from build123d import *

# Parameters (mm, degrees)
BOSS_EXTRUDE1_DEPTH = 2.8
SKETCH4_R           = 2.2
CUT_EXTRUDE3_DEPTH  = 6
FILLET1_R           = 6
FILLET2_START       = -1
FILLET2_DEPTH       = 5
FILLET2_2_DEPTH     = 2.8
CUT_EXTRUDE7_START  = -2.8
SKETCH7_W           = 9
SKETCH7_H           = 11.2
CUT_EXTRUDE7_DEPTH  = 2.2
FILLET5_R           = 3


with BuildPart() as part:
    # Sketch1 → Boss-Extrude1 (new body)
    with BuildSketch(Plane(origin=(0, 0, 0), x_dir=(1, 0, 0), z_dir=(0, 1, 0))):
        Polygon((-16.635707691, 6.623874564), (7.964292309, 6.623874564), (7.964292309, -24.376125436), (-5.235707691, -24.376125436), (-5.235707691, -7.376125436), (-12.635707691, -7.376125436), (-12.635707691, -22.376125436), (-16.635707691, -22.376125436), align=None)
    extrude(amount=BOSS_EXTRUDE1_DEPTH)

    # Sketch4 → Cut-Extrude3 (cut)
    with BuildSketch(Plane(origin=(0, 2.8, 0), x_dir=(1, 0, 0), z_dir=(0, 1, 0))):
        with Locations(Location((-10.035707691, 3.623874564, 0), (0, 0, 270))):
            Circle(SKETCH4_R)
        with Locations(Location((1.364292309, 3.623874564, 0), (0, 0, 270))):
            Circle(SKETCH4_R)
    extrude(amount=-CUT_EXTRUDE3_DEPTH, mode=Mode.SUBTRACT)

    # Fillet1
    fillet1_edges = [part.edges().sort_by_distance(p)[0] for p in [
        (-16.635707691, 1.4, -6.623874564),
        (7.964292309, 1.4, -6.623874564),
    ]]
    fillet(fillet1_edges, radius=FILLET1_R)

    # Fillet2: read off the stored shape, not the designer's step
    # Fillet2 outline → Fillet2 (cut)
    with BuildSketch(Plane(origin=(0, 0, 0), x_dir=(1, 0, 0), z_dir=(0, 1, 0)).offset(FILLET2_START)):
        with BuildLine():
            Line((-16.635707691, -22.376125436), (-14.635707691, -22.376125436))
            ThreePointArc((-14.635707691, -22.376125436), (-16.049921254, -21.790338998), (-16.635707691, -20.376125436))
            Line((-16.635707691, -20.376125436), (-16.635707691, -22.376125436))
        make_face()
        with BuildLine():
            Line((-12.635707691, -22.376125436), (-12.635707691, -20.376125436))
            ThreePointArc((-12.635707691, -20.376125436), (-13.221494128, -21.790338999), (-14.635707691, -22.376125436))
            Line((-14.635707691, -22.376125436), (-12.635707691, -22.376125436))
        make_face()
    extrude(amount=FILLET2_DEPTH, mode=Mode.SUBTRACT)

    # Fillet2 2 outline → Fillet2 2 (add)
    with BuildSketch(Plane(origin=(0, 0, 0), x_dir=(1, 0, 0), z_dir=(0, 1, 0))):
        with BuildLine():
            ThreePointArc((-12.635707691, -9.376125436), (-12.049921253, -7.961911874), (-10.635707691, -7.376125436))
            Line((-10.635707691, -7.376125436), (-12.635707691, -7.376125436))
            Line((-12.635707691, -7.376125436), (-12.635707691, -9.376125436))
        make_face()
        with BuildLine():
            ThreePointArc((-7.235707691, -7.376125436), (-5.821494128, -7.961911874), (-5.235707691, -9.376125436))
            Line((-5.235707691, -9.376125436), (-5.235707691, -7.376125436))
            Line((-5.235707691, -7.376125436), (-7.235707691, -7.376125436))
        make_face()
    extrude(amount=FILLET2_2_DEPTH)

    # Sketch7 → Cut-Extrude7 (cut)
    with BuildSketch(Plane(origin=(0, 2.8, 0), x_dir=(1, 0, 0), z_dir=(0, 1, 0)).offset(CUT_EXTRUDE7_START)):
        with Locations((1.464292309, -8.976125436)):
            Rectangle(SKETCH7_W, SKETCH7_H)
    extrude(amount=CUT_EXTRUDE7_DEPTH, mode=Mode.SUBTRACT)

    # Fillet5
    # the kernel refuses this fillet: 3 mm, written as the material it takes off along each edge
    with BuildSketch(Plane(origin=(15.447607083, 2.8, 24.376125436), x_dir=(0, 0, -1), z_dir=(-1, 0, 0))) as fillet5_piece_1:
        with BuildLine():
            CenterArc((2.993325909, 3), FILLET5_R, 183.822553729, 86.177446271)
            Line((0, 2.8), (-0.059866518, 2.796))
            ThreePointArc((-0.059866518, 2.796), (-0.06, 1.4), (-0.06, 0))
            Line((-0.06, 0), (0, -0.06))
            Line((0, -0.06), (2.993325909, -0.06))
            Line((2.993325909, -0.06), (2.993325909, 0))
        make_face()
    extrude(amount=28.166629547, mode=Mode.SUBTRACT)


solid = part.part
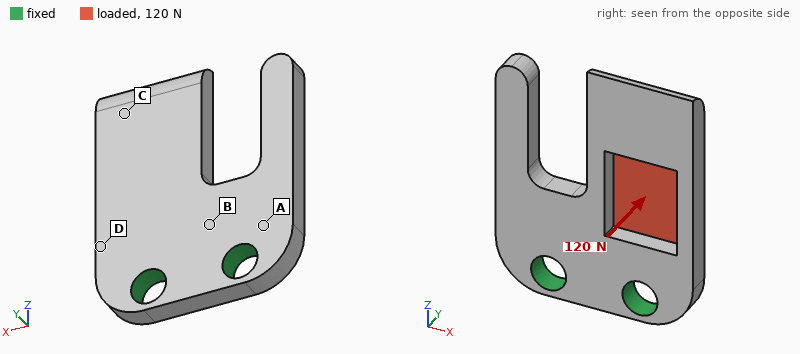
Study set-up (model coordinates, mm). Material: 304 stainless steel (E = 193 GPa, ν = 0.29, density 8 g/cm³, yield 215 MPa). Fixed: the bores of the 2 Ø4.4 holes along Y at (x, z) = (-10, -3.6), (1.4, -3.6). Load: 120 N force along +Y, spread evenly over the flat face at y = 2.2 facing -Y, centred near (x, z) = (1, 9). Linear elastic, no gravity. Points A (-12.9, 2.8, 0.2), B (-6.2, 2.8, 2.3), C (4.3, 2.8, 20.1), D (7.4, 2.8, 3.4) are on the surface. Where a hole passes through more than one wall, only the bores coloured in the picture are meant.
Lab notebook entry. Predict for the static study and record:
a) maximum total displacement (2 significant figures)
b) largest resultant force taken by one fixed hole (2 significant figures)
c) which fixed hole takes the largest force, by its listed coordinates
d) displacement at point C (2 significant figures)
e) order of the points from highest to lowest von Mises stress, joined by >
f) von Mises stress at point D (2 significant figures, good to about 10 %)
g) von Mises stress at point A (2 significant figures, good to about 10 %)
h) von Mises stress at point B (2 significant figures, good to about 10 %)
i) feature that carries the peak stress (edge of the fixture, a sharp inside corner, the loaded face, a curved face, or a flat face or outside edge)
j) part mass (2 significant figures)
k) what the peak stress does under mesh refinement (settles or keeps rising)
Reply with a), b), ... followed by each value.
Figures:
a) 46 µm
b) 110 N
c) (1.4, -3.6)
d) 35 µm
e) D > B > A > C
f) 53 MPa
g) 17 MPa
h) 30 MPa
i) edge of the fixture
j) 11 g
k) keeps rising
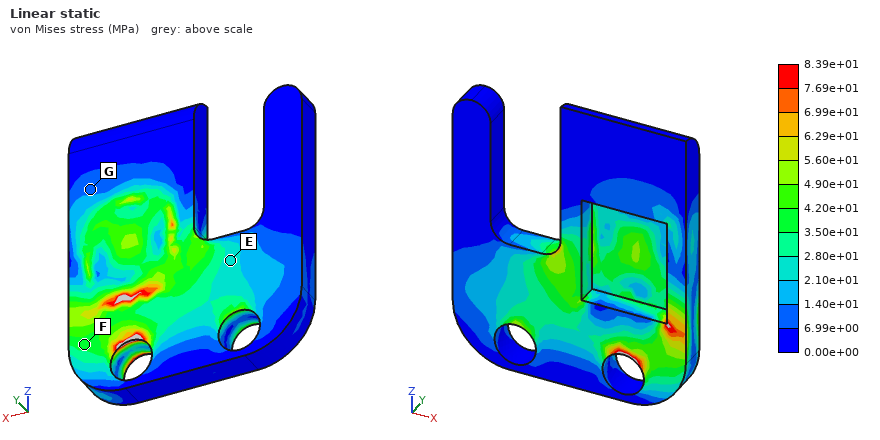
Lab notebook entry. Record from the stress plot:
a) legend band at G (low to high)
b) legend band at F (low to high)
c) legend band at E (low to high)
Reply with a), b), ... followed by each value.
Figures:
a) 6.99e+00 to 1.40e+01 MPa
b) 3.50e+01 to 4.20e+01 MPa
c) 2.10e+01 to 2.80e+01 MPa
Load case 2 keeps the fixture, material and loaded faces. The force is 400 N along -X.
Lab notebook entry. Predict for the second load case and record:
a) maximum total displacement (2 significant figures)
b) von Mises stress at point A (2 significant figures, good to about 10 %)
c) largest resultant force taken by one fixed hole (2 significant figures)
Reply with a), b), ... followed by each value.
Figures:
a) 8.7 µm
b) 10 MPa
c) 370 N
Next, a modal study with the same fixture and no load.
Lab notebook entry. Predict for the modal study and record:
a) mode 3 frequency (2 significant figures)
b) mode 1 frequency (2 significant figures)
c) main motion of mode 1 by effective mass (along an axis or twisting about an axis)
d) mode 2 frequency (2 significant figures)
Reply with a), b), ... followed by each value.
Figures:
a) 9300 Hz
b) 3100 Hz
c) along Y
d) 5400 Hz
